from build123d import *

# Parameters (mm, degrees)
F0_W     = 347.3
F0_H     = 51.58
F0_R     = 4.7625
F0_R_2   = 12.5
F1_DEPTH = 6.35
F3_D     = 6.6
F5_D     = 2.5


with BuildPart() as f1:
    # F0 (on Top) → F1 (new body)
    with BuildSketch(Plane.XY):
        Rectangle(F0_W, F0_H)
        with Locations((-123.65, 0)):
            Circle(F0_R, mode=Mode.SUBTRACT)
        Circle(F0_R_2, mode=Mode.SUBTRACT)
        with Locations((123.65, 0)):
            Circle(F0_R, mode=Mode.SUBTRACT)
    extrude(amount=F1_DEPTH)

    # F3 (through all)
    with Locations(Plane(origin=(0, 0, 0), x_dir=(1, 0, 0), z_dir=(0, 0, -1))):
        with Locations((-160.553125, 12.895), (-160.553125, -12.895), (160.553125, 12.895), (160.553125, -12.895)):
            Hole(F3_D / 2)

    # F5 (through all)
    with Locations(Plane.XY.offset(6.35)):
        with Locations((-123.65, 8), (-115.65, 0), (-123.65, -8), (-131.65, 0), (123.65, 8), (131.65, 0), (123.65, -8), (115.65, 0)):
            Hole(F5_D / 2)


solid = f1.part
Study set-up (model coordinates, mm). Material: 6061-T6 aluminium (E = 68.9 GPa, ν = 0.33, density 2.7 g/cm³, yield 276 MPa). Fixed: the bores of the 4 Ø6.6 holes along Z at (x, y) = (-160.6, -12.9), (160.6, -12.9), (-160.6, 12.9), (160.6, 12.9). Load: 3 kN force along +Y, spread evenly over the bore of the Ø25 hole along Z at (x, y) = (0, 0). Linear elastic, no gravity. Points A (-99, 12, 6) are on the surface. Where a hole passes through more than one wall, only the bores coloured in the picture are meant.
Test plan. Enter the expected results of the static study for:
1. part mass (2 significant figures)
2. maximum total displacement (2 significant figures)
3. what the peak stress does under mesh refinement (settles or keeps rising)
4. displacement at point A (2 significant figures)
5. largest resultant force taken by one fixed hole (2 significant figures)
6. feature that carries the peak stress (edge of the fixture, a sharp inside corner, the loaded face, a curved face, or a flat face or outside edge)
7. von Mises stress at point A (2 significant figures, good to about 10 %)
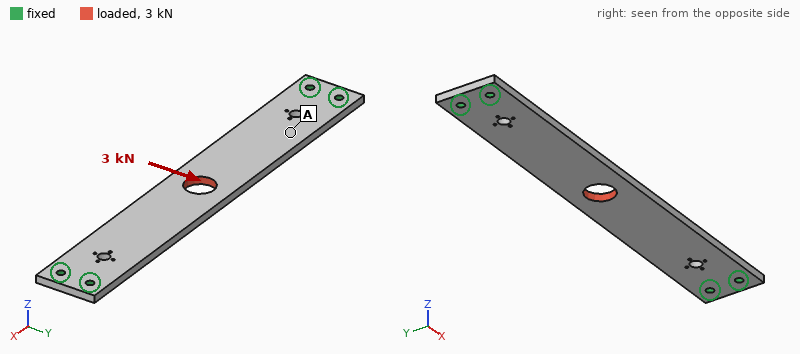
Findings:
290 g
0.15 mm
keeps rising
0.059 mm
3.9 kN
edge of the fixture
10 MPa
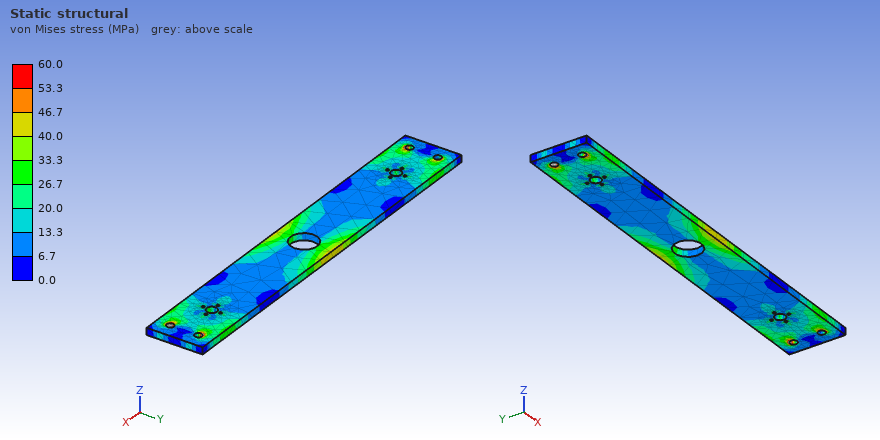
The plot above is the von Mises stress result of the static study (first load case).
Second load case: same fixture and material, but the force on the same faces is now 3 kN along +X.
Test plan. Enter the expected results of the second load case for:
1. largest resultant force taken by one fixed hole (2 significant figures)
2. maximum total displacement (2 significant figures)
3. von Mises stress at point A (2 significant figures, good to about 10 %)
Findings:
750 N
11 µm
4.6 MPa
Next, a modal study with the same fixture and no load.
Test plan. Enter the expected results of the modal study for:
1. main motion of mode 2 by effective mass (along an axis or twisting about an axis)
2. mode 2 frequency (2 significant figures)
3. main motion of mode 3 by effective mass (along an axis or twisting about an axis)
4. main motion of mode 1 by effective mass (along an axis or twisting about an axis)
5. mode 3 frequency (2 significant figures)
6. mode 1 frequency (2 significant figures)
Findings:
twisting about Y
890 Hz
twisting about X
along Z
1200 Hz
320 Hz
